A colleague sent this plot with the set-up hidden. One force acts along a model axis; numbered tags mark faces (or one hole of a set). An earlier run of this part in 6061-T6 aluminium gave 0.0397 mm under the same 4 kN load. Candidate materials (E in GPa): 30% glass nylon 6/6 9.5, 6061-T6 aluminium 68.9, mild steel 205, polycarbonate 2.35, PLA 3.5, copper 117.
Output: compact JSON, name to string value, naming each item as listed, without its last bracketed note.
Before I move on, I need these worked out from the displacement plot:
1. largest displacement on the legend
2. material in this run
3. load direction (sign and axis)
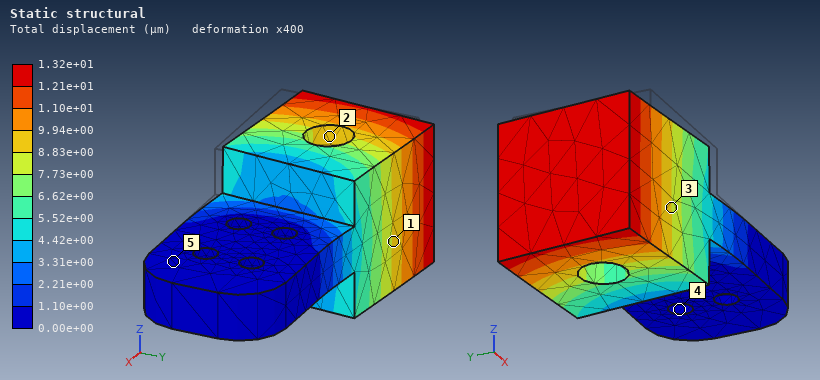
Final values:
{"largest displacement on the legend": "1.32e+01 µm", "material in this run": "mild steel", "load direction": "+Y"}
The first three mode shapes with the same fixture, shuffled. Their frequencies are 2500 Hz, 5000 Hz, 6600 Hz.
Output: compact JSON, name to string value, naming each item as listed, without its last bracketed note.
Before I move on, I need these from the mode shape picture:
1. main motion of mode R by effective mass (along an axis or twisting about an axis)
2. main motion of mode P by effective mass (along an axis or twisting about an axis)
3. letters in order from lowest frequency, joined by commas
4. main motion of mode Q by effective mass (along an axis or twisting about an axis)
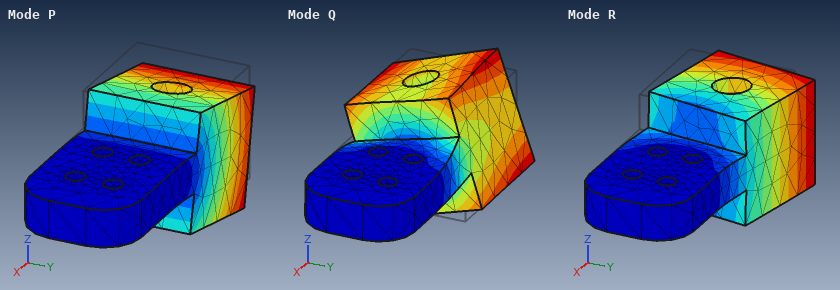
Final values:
{"main motion of mode R by effective mass": "along Y", "main motion of mode P by effective mass": "along Z", "letters in order from lowest frequency, joined by commas": "P, R, Q", "main motion of mode Q by effective mass": "twisting about X"}
